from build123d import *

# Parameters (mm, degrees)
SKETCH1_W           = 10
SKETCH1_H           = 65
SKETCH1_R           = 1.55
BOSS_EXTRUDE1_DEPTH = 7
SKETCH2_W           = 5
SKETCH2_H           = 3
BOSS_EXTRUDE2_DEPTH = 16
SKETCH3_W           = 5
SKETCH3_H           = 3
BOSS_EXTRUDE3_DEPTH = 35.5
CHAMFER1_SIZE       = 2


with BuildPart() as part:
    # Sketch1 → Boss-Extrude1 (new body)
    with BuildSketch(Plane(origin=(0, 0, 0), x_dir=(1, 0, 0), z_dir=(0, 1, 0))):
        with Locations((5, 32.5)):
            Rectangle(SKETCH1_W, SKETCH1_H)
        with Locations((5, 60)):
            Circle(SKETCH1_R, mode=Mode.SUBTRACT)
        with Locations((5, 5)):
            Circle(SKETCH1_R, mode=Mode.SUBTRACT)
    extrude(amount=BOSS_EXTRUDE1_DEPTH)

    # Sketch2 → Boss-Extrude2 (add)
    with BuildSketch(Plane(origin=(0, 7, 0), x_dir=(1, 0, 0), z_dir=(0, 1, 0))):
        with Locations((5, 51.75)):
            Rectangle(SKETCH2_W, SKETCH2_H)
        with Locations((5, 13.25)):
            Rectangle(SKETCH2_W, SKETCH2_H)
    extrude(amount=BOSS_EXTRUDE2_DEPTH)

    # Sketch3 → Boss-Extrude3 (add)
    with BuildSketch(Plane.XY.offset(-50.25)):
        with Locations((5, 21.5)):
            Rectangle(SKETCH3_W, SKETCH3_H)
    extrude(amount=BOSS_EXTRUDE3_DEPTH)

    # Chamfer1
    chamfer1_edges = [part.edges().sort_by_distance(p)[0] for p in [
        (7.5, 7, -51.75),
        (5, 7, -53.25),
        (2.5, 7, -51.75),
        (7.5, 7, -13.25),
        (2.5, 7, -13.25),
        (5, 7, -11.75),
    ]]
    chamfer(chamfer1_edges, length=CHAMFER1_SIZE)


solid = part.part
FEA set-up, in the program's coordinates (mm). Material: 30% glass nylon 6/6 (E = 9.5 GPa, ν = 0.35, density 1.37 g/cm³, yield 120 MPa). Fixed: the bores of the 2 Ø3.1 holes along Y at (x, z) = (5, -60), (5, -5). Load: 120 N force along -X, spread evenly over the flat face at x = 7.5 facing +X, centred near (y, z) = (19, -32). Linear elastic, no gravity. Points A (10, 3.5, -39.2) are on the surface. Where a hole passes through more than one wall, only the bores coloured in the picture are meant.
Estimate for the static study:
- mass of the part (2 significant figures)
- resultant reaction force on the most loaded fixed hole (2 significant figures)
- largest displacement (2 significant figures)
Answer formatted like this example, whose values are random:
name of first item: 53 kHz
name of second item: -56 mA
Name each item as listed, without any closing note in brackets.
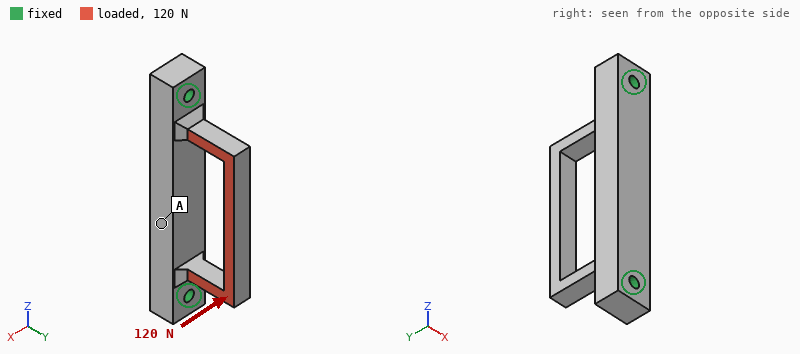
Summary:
mass of the part: 7.6 g
resultant reaction force on the most loaded fixed hole: 60 N
largest displacement: 0.36 mm
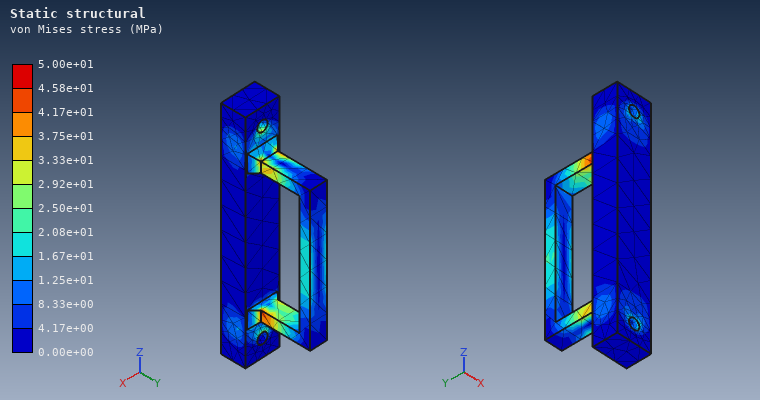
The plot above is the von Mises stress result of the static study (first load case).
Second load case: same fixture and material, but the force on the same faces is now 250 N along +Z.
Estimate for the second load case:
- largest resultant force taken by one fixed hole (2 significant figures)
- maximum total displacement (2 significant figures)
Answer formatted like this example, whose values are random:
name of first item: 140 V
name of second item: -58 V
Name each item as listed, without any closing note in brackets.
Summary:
largest resultant force taken by one fixed hole: 140 N
maximum total displacement: 0.46 mm
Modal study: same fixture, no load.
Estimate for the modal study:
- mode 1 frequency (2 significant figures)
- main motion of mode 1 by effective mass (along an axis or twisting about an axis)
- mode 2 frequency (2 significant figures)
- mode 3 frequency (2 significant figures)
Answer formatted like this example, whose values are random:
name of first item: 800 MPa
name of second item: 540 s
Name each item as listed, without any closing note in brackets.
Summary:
mode 1 frequency: 2900 Hz
main motion of mode 1 by effective mass: along X
mode 2 frequency: 3500 Hz
mode 3 frequency: 4400 Hz
